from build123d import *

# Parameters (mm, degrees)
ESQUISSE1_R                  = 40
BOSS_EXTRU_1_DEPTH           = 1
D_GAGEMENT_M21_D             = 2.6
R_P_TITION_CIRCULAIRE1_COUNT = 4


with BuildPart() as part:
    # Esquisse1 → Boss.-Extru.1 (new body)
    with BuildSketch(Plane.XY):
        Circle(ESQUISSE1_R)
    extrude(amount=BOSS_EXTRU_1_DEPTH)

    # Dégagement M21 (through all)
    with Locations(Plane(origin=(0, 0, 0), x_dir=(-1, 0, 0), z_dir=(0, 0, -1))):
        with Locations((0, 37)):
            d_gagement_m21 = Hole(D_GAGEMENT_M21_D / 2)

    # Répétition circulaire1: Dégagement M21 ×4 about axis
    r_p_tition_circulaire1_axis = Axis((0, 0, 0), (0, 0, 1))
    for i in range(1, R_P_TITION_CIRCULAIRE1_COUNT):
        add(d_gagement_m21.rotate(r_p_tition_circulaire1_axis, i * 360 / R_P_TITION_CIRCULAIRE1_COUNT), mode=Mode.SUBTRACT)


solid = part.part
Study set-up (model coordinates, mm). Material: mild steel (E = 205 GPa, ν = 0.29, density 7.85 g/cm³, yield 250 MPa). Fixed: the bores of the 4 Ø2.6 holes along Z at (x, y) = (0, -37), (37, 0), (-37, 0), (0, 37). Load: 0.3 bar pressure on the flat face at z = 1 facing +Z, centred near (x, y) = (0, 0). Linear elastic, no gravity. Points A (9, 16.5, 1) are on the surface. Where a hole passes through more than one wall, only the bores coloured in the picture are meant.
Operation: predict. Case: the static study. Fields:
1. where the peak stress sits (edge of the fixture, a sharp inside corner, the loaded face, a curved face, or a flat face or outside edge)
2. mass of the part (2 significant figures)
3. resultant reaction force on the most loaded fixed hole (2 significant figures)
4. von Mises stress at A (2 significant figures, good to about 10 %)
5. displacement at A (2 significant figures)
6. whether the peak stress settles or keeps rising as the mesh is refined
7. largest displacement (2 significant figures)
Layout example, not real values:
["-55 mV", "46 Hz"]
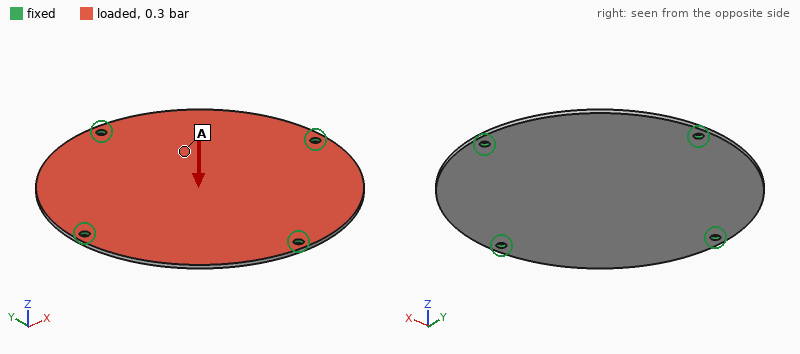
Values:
["edge of the fixture", "39 g", "38 N", "22 MPa", "60 µm", "keeps rising", "84 µm"]
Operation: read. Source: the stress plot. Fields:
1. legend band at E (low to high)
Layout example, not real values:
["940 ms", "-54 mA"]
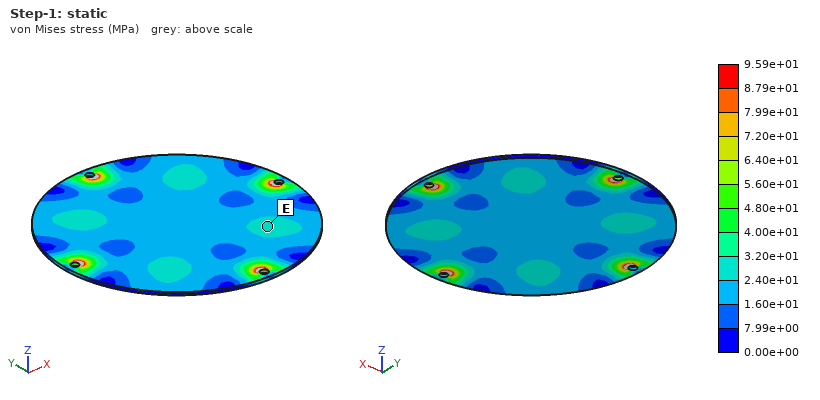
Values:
["2.40e+01 to 3.20e+01 MPa"]
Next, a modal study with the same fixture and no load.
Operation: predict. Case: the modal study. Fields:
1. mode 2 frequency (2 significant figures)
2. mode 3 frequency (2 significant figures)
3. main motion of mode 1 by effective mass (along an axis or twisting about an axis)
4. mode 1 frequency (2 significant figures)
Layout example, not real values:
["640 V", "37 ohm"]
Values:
["1700 Hz", "1700 Hz", "along Z", "1300 Hz"]
